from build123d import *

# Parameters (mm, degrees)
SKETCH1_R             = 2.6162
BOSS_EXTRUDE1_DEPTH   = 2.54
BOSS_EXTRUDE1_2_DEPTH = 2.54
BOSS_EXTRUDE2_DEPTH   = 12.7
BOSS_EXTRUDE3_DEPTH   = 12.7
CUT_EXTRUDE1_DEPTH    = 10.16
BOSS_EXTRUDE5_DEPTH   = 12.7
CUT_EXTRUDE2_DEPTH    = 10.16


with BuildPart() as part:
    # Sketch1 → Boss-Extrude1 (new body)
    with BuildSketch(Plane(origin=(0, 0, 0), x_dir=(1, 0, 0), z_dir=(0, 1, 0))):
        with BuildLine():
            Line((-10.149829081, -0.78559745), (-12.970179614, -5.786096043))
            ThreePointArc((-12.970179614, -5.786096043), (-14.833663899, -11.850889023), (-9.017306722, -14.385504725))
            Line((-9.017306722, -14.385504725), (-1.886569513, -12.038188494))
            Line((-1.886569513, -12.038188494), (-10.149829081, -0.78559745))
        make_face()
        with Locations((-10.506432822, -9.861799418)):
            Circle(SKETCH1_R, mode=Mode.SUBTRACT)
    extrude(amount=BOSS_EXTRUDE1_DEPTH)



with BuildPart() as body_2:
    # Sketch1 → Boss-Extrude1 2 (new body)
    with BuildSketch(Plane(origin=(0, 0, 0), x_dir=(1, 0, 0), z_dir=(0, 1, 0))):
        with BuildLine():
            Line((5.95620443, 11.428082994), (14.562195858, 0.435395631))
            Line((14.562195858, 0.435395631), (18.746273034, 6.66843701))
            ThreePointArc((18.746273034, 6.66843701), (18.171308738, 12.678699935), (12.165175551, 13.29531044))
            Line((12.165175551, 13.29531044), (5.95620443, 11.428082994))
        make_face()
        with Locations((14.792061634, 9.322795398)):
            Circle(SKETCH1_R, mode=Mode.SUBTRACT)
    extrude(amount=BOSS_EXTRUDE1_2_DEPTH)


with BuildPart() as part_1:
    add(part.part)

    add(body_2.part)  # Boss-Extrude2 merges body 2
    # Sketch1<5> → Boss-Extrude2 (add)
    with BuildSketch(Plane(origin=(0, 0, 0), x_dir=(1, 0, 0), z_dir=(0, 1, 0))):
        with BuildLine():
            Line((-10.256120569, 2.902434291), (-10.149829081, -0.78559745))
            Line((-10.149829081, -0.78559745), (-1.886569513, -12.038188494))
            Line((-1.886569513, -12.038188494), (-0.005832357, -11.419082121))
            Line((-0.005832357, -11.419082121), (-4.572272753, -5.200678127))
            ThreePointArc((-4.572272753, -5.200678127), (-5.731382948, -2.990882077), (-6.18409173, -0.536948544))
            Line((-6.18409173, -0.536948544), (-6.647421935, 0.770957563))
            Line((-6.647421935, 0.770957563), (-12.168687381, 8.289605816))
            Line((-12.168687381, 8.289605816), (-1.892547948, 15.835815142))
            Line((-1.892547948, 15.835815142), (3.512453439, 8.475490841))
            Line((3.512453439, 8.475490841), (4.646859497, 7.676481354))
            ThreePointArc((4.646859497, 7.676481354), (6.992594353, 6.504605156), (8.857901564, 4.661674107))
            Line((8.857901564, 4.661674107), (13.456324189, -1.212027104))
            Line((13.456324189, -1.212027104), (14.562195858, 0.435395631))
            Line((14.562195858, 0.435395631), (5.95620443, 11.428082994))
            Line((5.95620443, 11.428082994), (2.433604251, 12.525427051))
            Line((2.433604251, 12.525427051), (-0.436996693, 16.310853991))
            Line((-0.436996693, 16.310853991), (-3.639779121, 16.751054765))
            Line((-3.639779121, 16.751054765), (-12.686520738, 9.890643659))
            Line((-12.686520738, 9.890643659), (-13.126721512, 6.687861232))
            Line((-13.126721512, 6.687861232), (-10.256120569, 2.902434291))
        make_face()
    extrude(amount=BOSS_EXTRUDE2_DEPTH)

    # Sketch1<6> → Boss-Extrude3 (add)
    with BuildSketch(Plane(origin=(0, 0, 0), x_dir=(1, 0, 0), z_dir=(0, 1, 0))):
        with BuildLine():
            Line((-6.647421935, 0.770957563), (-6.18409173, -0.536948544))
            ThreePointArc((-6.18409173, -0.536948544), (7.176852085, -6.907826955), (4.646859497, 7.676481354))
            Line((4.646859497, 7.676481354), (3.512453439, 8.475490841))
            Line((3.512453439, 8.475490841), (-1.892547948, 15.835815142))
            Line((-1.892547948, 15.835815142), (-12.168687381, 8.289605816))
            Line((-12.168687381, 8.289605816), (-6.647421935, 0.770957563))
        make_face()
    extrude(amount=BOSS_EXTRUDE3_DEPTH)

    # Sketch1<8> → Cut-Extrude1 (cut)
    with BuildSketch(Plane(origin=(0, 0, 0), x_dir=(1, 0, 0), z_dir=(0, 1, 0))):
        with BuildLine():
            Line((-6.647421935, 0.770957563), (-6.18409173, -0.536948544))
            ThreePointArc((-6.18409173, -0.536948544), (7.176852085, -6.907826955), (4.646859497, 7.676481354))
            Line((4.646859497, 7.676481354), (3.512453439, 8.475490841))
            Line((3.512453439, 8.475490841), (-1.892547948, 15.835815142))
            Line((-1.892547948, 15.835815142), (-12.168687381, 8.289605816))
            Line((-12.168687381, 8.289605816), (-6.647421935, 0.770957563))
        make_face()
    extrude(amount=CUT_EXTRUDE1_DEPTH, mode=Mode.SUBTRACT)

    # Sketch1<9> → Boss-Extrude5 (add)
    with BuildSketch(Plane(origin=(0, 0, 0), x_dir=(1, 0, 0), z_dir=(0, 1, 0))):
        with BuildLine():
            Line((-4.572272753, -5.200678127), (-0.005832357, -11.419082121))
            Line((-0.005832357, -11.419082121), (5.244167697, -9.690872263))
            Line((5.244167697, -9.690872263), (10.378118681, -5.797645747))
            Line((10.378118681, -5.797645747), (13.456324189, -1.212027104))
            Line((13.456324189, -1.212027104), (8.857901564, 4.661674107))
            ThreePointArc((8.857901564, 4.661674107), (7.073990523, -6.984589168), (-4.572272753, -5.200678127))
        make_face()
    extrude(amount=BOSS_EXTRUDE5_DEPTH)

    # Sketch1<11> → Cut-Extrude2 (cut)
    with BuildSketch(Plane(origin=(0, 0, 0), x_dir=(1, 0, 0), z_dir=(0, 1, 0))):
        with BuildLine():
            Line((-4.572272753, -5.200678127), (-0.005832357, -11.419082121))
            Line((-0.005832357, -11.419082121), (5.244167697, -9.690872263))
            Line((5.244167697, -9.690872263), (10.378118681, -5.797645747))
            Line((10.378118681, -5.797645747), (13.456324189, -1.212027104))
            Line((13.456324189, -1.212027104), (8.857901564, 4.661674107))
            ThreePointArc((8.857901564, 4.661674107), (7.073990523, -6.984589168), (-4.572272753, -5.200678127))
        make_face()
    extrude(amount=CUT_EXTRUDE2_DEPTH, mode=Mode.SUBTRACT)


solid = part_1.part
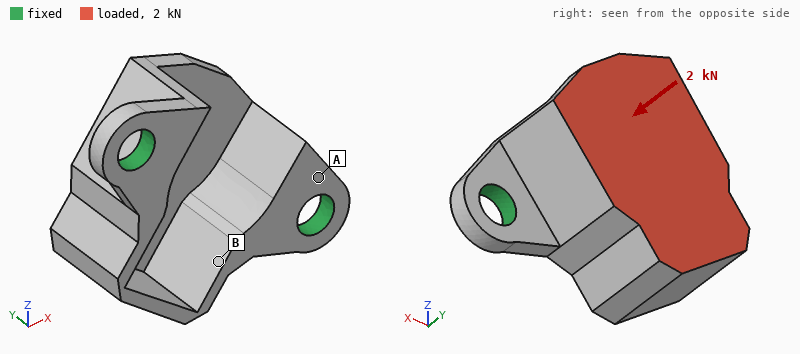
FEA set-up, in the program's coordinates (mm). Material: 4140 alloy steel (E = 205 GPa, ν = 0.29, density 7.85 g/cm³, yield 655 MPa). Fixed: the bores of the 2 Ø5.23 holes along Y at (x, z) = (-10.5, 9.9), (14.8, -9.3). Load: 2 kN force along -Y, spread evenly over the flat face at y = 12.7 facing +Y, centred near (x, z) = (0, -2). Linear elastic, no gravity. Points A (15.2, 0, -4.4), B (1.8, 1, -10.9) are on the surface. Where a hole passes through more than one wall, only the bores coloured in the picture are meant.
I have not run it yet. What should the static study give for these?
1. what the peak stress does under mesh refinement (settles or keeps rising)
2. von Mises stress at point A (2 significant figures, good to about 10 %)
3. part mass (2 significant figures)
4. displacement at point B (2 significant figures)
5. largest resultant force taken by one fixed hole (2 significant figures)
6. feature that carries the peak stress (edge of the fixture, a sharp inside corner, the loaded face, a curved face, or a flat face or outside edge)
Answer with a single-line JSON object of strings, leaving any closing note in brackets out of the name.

{"what the peak stress does under mesh refinement": "keeps rising", "von Mises stress at point A": "81 MPa", "part mass": "22 g", "displacement at point B": "29 µm", "largest resultant force taken by one fixed hole": "1.1 kN", "feature that carries the peak stress": "edge of the fixture"}
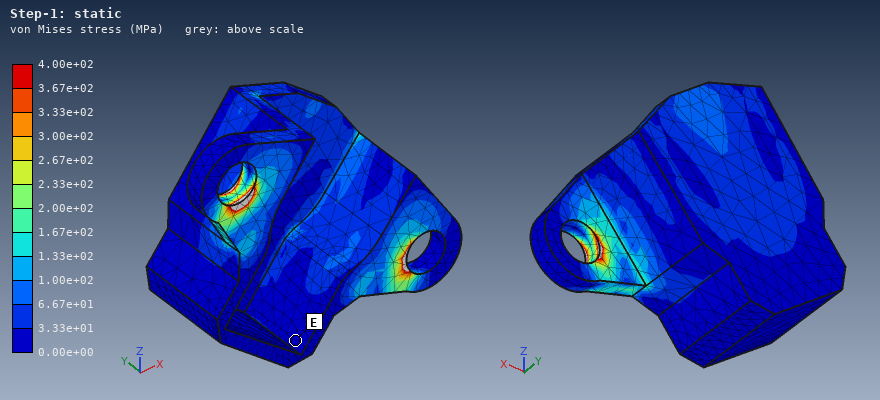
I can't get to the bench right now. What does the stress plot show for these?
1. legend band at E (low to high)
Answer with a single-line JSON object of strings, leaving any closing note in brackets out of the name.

{"legend band at E": "0.00e+00 to 3.33e+01 MPa"}
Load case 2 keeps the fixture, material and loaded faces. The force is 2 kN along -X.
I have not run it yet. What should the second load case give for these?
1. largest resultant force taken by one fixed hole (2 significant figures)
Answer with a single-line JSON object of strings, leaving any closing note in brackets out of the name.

{"largest resultant force taken by one fixed hole": "1.3 kN"}
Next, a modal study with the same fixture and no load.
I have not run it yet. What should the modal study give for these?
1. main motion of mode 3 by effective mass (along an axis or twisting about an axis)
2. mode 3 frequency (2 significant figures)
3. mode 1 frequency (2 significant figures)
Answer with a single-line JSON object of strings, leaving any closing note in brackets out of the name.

{"main motion of mode 3 by effective mass": "twisting about Y", "mode 3 frequency": "11 kHz", "mode 1 frequency": "5200 Hz"}
